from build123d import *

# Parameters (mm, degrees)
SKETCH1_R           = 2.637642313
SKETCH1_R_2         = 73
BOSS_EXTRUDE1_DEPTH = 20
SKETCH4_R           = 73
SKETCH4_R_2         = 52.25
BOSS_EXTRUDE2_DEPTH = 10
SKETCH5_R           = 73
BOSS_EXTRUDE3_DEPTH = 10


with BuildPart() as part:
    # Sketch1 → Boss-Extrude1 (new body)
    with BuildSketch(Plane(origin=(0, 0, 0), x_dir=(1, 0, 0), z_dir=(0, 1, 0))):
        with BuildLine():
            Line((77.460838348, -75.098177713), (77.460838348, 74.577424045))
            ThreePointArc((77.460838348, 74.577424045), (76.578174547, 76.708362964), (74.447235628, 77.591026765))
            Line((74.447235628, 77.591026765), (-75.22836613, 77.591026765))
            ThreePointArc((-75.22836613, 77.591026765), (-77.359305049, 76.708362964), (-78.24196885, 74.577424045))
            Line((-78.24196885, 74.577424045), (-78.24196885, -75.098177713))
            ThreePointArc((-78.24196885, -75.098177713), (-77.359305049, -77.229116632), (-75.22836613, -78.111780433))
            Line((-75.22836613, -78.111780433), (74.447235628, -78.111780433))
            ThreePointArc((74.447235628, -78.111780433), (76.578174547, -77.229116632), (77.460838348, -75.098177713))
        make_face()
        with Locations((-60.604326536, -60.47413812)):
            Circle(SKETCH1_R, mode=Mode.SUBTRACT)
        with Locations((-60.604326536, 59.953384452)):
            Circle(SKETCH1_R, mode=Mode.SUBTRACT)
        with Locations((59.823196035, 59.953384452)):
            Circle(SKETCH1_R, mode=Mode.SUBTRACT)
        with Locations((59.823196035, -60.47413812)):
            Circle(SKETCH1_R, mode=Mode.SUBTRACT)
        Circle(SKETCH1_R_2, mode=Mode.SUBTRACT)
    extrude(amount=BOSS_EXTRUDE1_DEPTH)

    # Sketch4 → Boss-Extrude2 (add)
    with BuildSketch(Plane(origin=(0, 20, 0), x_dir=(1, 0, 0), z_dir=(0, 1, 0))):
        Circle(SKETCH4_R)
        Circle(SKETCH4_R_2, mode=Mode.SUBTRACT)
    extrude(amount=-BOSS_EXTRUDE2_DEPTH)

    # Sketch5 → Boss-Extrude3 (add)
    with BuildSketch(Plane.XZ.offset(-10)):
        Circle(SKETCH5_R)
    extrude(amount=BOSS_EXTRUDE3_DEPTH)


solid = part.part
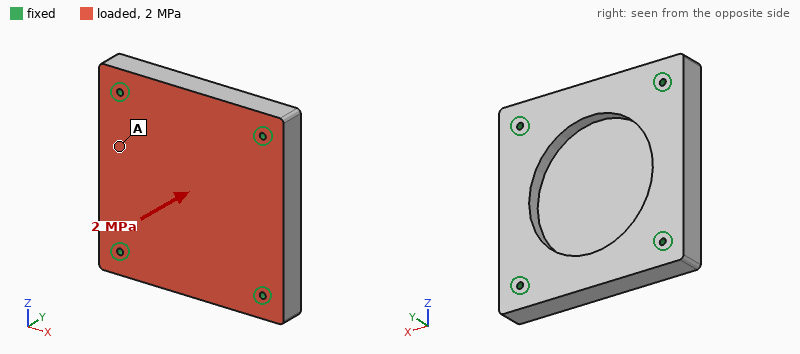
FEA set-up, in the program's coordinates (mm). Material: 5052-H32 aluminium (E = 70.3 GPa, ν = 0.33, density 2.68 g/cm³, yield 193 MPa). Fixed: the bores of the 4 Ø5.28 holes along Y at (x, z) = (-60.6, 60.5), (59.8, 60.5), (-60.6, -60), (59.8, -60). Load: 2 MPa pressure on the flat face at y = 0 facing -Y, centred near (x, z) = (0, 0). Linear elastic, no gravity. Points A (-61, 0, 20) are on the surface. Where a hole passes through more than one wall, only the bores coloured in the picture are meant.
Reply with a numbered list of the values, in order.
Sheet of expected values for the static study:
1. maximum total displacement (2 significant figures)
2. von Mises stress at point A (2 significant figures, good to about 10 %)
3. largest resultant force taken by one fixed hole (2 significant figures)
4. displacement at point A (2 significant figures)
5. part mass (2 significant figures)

1. 0.17 mm
2. 23 MPa
3. 13 kN
4. 0.060 mm
5. 1.1 kg
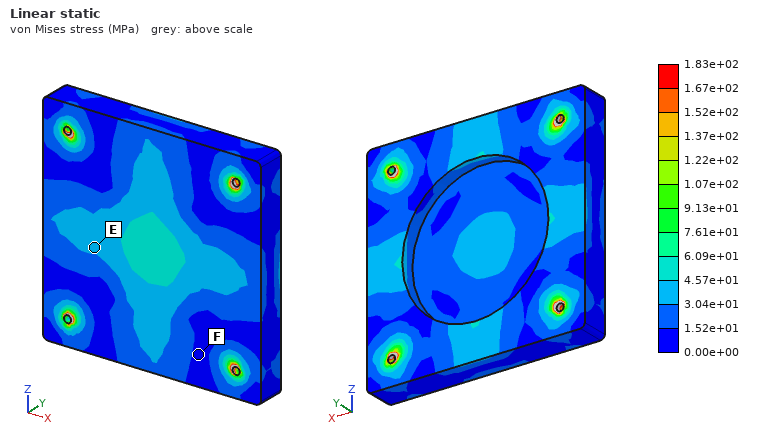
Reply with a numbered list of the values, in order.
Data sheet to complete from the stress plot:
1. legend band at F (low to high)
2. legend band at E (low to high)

1. 0.00e+00 to 1.52e+01 MPa
2. 3.04e+01 to 4.57e+01 MPa
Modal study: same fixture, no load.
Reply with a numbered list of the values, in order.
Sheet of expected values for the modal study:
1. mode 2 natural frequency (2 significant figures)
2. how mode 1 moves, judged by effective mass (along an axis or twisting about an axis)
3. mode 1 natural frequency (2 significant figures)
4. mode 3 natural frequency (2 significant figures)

1. 5600 Hz
2. along Y
3. 3900 Hz
4. 5600 Hz
